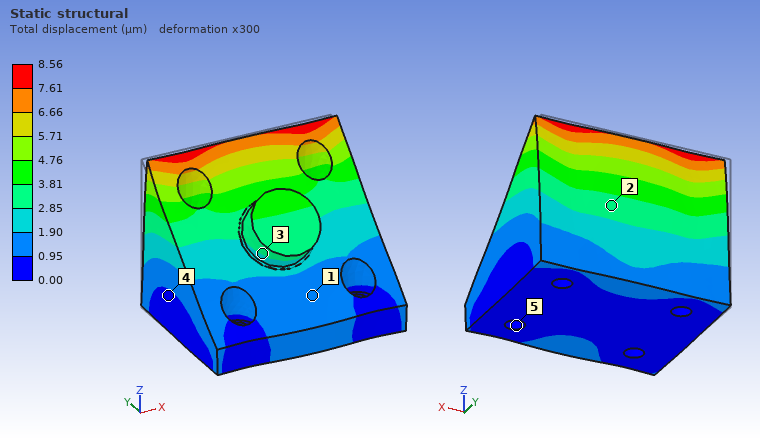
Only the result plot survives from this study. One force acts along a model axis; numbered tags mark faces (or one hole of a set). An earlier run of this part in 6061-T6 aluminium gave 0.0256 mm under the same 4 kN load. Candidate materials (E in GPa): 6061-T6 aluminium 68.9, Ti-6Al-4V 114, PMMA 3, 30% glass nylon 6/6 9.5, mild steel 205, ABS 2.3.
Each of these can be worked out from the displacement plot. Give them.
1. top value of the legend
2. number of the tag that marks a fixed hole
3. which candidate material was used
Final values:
8.56 µm
5
mild steel
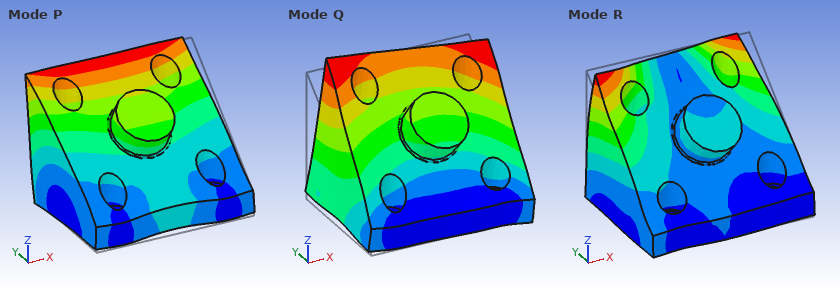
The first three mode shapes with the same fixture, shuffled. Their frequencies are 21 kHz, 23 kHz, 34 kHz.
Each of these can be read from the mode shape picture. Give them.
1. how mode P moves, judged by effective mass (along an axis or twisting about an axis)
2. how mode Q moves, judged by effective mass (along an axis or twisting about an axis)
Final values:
along Y
along X
